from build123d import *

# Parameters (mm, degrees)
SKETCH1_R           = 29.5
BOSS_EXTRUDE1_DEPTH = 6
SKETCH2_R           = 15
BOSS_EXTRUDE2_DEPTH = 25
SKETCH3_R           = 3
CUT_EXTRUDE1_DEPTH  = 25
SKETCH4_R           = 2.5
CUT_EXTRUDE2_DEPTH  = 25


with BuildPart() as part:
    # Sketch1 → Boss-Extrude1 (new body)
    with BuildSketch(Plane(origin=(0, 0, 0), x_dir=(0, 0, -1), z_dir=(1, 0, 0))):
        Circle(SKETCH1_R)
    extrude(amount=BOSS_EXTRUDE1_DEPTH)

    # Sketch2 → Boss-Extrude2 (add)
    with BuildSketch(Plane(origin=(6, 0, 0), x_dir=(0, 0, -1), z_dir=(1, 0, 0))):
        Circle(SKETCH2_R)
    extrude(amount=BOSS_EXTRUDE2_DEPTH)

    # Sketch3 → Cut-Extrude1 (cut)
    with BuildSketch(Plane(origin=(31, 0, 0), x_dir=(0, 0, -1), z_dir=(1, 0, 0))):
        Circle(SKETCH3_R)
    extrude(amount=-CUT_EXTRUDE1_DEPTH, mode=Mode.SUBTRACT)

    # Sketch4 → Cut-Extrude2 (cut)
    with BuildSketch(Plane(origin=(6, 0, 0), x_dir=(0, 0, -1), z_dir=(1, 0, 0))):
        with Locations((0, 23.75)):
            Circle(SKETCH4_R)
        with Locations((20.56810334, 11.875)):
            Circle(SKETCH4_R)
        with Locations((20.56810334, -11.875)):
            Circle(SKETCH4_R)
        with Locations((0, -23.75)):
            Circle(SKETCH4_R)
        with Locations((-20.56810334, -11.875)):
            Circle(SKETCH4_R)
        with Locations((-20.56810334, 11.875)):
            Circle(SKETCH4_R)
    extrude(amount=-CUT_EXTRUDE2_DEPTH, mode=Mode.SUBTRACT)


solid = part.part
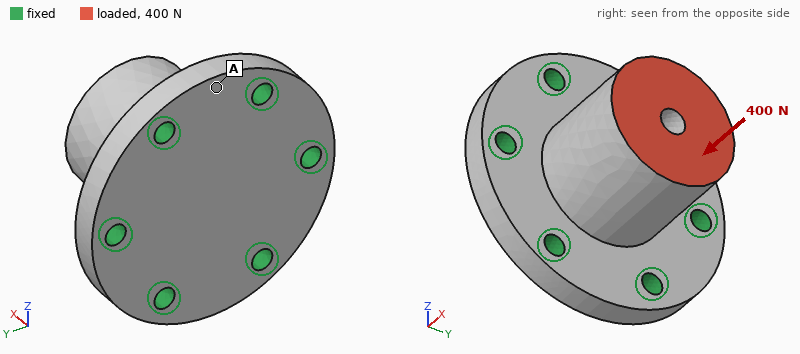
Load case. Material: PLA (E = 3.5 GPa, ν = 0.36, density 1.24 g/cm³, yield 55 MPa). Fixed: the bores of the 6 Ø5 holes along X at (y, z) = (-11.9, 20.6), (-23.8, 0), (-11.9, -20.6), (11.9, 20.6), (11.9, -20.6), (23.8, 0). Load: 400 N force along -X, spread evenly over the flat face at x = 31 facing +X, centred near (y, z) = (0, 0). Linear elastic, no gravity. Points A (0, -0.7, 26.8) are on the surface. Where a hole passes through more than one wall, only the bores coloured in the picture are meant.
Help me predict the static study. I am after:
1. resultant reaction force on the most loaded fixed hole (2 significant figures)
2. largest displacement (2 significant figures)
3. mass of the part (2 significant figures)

71 N
17 µm
41 g
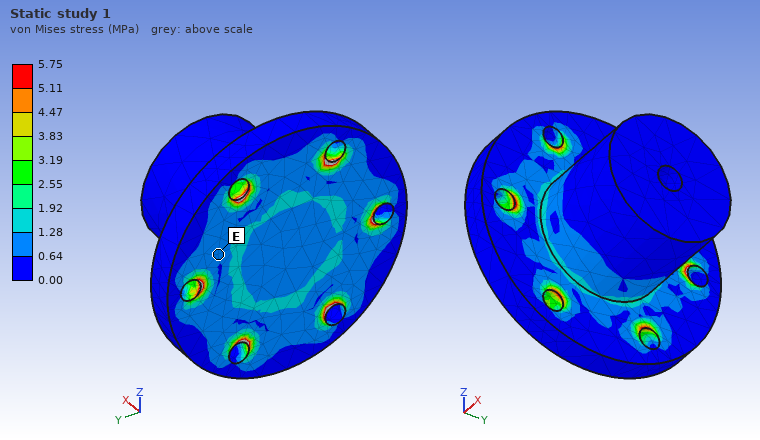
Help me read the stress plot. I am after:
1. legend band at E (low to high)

0.64 to 1.28 MPa
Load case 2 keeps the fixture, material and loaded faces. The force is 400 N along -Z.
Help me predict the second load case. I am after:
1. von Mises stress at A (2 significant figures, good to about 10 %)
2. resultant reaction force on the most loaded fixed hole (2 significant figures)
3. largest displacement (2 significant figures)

1.6 MPa
190 N
91 µm
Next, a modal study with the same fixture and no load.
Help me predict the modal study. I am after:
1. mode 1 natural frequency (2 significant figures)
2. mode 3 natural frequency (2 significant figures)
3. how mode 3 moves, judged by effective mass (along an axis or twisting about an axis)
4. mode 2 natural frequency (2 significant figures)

3800 Hz
5100 Hz
along X
3800 Hz
